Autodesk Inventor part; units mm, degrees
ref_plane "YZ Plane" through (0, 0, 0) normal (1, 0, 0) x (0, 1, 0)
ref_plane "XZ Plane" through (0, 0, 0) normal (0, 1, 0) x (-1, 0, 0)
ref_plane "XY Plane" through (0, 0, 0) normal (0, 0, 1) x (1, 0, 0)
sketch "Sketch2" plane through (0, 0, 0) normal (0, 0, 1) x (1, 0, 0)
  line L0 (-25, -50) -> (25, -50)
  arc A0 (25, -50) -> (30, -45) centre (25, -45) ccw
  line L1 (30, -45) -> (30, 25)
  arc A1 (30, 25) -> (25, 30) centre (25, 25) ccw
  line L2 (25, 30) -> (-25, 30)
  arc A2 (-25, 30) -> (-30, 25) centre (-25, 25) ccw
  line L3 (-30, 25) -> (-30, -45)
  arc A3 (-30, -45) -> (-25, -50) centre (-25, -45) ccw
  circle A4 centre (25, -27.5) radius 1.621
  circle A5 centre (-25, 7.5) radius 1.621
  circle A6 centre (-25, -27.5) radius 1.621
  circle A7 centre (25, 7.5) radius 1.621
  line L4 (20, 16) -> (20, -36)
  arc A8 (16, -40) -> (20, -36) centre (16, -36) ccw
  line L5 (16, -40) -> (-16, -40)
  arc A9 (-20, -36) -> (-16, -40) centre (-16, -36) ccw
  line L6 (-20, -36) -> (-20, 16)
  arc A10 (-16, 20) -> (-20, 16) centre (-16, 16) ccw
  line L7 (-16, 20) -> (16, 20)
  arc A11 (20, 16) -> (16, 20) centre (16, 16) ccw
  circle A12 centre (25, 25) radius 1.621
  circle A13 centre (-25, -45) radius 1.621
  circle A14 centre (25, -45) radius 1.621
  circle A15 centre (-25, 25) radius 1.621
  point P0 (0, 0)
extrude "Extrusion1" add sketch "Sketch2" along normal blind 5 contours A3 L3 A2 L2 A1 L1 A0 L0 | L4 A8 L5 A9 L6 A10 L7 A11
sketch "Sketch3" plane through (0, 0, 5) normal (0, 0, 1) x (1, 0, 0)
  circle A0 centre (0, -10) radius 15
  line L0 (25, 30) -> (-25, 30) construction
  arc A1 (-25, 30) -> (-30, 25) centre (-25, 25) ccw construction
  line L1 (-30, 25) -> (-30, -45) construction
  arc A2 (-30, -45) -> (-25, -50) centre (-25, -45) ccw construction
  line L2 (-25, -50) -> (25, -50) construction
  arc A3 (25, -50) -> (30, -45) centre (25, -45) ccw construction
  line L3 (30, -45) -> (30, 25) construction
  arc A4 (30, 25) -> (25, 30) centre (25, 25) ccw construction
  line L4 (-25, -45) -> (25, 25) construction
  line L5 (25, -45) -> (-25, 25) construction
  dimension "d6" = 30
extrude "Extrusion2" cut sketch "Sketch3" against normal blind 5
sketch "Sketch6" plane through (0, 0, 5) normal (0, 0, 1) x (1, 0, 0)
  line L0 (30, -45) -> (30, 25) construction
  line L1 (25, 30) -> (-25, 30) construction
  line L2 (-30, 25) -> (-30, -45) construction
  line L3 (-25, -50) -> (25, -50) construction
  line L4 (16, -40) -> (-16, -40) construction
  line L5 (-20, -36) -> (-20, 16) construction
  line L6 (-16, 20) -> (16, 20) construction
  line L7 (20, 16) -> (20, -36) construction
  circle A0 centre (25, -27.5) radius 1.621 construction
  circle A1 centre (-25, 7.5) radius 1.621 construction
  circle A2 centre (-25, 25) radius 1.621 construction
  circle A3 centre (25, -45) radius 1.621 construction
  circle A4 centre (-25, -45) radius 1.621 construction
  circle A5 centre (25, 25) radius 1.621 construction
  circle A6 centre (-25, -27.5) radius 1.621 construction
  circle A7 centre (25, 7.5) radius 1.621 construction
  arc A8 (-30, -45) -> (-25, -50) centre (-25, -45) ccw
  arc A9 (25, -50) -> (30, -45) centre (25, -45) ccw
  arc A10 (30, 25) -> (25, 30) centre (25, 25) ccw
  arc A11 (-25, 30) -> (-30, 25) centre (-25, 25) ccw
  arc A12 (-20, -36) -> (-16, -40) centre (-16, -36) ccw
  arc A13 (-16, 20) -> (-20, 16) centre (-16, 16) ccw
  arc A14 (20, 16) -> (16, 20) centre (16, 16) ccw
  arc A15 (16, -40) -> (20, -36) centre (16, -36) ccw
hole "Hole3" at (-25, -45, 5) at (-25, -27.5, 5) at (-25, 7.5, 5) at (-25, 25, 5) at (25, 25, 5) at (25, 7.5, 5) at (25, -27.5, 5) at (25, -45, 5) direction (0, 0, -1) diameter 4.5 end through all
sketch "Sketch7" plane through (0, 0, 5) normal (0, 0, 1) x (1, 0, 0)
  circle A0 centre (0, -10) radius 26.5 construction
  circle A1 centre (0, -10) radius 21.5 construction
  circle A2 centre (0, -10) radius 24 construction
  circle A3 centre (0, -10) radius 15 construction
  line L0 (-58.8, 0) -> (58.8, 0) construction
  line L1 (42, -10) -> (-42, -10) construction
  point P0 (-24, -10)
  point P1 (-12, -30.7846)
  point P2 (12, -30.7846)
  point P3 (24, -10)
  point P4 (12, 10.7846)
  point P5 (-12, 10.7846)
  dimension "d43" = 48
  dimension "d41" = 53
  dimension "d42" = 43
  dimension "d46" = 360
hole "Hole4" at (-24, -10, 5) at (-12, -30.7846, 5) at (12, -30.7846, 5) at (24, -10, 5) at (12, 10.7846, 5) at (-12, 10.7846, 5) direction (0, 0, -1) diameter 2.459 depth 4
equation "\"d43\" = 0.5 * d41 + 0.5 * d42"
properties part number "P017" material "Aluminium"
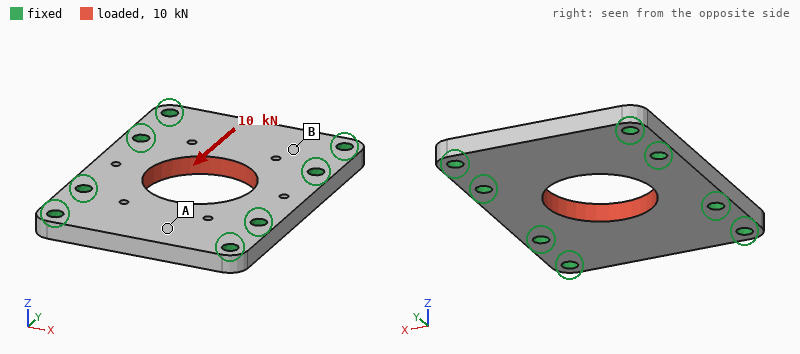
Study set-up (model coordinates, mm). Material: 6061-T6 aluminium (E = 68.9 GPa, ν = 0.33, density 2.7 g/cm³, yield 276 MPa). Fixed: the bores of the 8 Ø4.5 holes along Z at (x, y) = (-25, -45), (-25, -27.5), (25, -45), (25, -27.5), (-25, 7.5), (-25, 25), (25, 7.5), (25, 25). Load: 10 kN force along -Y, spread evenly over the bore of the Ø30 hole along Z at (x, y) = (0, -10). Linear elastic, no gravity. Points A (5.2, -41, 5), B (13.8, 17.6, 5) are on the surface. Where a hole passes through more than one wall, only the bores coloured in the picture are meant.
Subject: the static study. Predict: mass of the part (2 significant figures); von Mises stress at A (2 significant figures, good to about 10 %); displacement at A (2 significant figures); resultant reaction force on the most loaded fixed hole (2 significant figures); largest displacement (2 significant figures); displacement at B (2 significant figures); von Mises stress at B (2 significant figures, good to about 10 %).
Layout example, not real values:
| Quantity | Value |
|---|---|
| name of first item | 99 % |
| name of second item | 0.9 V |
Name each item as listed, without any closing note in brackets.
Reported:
| Quantity | Value |
|---|---|
| mass of the part | 53 g |
| von Mises stress at A | 11 MPa |
| displacement at A | 8.5 µm |
| resultant reaction force on the most loaded fixed hole | 1.7 kN |
| largest displacement | 12 µm |
| displacement at B | 5.4 µm |
| von Mises stress at B | 22 MPa |
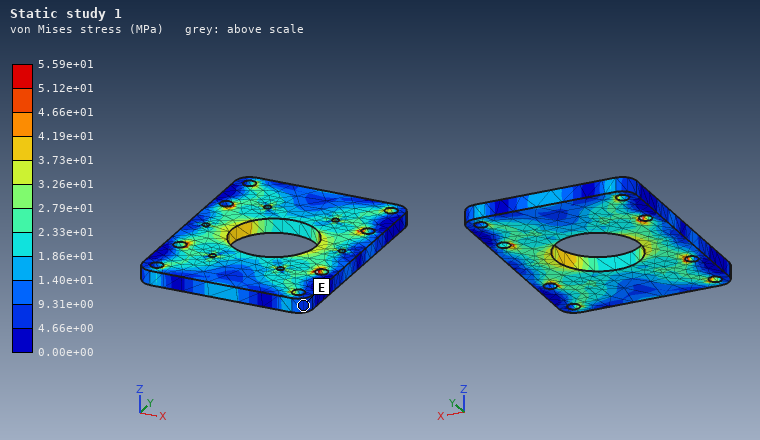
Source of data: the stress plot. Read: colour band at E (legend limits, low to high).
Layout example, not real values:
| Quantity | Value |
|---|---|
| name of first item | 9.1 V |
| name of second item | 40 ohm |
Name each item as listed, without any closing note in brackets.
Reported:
| Quantity | Value |
|---|---|
| colour band at E | 4.66e+00 to 9.31e+00 MPa |
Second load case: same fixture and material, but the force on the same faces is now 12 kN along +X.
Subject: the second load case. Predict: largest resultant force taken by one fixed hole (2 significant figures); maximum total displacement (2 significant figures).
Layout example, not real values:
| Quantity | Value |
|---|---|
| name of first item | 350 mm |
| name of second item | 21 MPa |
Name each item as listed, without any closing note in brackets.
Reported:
| Quantity | Value |
|---|---|
| largest resultant force taken by one fixed hole | 2.6 kN |
| maximum total displacement | 15 µm |
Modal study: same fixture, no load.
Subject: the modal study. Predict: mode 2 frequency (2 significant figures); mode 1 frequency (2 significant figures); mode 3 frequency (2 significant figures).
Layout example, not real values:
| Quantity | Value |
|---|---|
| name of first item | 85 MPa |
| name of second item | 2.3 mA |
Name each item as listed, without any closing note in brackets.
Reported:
| Quantity | Value |
|---|---|
| mode 2 frequency | 11 kHz |
| mode 1 frequency | 11 kHz |
| mode 3 frequency | 15 kHz |
